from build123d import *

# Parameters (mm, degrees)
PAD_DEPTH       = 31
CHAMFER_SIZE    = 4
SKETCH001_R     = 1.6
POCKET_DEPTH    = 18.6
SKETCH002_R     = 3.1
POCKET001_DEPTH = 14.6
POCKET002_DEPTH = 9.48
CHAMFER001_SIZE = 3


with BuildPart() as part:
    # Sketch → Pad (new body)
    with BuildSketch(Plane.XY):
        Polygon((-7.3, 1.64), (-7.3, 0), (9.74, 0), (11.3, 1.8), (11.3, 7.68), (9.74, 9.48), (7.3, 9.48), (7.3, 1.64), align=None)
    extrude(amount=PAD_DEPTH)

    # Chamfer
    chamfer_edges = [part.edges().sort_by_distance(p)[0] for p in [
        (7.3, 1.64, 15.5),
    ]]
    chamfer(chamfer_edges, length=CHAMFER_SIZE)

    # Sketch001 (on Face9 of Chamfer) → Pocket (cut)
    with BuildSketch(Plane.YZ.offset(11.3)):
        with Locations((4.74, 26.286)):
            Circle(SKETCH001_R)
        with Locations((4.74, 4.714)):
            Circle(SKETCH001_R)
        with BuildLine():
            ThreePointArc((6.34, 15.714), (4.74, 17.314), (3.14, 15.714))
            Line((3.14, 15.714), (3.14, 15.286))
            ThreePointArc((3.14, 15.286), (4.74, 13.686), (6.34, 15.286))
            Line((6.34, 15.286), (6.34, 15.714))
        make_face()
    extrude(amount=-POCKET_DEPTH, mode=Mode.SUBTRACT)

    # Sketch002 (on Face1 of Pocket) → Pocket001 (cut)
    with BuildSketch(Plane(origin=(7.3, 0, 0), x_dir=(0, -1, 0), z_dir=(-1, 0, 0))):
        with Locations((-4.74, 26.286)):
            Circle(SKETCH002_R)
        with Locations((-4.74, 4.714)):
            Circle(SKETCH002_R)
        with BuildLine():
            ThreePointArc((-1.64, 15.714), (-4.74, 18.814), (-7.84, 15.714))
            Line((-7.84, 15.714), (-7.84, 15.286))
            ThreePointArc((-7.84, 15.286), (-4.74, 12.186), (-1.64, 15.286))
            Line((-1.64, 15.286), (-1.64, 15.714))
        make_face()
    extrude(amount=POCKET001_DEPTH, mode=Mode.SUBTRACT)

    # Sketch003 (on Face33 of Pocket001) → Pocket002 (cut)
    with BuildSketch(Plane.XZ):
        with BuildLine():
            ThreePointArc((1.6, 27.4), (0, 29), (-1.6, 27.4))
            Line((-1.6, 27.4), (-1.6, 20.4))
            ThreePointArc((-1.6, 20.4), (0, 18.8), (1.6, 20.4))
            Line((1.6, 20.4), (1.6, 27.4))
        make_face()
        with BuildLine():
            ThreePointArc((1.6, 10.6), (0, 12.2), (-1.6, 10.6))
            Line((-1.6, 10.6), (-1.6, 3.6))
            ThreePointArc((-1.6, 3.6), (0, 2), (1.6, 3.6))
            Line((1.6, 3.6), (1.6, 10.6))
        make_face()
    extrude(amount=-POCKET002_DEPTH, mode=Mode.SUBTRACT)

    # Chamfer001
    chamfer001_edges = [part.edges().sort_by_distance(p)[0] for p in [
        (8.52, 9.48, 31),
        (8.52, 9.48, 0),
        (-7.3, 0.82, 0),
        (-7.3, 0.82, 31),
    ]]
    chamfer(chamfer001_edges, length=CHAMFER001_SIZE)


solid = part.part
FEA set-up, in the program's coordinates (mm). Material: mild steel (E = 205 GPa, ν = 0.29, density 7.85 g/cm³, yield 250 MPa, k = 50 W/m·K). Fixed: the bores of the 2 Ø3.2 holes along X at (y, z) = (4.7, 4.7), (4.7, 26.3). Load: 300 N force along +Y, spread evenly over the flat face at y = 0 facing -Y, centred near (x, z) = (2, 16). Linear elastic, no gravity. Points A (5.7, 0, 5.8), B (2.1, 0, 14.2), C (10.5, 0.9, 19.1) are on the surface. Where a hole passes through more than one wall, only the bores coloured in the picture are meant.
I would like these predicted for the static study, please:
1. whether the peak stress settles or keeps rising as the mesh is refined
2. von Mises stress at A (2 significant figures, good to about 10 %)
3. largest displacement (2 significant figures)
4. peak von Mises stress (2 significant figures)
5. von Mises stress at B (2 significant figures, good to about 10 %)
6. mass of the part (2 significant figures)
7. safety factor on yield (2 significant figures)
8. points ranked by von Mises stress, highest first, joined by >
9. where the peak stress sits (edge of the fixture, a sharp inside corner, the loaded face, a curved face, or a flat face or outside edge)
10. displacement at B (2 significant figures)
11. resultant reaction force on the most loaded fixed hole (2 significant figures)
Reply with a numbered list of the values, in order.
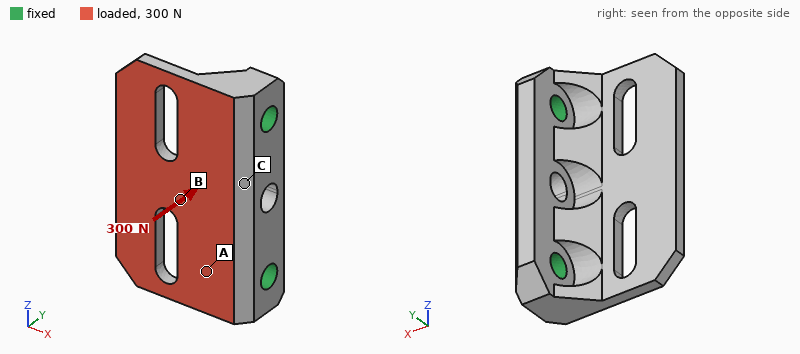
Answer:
1. settles
2. 22 MPa
3. 46 µm
4. 170 MPa
5. 110 MPa
6. 14 g
7. 1.5
8. B > A > C
9. the loaded face
10. 7.2 µm
11. 150 N
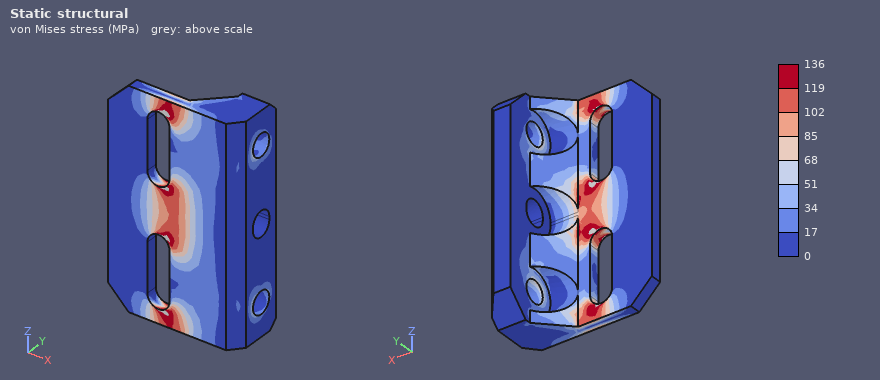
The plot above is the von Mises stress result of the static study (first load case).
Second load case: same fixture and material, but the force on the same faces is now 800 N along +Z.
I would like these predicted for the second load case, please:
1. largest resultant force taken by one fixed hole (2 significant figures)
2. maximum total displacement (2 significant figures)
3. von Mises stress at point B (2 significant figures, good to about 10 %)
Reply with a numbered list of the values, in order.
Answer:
1. 490 N
2. 5.9 µm
3. 29 MPa
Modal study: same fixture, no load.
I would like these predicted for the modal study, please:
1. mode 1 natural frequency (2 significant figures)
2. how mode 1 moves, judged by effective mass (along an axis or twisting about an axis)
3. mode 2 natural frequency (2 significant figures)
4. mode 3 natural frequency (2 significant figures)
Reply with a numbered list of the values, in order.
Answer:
1. 6500 Hz
2. along Y
3. 11 kHz
4. 19 kHz
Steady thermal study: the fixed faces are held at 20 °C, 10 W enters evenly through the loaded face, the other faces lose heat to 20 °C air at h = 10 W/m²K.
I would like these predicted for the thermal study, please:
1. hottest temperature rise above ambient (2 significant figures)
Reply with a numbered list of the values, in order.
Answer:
1. 47 K
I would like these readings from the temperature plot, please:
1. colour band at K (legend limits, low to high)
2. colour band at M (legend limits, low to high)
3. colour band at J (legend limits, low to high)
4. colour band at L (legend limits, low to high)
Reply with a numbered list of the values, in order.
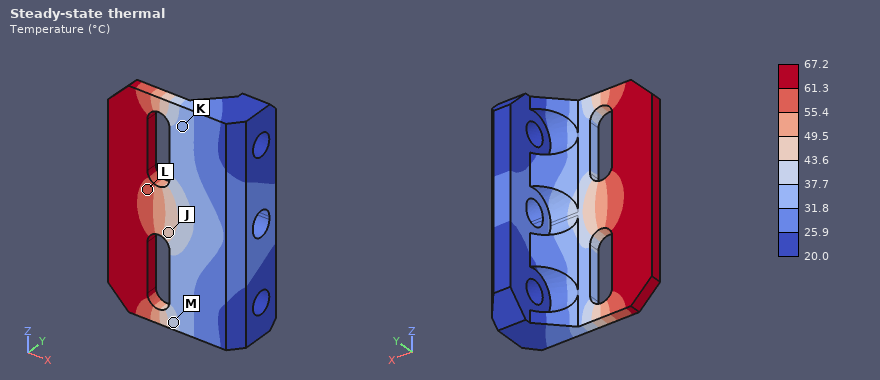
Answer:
1. 31.8 to 37.7 °C
2. 37.7 to 43.6 °C
3. 43.6 to 49.5 °C
4. 55.4 to 61.3 °C
